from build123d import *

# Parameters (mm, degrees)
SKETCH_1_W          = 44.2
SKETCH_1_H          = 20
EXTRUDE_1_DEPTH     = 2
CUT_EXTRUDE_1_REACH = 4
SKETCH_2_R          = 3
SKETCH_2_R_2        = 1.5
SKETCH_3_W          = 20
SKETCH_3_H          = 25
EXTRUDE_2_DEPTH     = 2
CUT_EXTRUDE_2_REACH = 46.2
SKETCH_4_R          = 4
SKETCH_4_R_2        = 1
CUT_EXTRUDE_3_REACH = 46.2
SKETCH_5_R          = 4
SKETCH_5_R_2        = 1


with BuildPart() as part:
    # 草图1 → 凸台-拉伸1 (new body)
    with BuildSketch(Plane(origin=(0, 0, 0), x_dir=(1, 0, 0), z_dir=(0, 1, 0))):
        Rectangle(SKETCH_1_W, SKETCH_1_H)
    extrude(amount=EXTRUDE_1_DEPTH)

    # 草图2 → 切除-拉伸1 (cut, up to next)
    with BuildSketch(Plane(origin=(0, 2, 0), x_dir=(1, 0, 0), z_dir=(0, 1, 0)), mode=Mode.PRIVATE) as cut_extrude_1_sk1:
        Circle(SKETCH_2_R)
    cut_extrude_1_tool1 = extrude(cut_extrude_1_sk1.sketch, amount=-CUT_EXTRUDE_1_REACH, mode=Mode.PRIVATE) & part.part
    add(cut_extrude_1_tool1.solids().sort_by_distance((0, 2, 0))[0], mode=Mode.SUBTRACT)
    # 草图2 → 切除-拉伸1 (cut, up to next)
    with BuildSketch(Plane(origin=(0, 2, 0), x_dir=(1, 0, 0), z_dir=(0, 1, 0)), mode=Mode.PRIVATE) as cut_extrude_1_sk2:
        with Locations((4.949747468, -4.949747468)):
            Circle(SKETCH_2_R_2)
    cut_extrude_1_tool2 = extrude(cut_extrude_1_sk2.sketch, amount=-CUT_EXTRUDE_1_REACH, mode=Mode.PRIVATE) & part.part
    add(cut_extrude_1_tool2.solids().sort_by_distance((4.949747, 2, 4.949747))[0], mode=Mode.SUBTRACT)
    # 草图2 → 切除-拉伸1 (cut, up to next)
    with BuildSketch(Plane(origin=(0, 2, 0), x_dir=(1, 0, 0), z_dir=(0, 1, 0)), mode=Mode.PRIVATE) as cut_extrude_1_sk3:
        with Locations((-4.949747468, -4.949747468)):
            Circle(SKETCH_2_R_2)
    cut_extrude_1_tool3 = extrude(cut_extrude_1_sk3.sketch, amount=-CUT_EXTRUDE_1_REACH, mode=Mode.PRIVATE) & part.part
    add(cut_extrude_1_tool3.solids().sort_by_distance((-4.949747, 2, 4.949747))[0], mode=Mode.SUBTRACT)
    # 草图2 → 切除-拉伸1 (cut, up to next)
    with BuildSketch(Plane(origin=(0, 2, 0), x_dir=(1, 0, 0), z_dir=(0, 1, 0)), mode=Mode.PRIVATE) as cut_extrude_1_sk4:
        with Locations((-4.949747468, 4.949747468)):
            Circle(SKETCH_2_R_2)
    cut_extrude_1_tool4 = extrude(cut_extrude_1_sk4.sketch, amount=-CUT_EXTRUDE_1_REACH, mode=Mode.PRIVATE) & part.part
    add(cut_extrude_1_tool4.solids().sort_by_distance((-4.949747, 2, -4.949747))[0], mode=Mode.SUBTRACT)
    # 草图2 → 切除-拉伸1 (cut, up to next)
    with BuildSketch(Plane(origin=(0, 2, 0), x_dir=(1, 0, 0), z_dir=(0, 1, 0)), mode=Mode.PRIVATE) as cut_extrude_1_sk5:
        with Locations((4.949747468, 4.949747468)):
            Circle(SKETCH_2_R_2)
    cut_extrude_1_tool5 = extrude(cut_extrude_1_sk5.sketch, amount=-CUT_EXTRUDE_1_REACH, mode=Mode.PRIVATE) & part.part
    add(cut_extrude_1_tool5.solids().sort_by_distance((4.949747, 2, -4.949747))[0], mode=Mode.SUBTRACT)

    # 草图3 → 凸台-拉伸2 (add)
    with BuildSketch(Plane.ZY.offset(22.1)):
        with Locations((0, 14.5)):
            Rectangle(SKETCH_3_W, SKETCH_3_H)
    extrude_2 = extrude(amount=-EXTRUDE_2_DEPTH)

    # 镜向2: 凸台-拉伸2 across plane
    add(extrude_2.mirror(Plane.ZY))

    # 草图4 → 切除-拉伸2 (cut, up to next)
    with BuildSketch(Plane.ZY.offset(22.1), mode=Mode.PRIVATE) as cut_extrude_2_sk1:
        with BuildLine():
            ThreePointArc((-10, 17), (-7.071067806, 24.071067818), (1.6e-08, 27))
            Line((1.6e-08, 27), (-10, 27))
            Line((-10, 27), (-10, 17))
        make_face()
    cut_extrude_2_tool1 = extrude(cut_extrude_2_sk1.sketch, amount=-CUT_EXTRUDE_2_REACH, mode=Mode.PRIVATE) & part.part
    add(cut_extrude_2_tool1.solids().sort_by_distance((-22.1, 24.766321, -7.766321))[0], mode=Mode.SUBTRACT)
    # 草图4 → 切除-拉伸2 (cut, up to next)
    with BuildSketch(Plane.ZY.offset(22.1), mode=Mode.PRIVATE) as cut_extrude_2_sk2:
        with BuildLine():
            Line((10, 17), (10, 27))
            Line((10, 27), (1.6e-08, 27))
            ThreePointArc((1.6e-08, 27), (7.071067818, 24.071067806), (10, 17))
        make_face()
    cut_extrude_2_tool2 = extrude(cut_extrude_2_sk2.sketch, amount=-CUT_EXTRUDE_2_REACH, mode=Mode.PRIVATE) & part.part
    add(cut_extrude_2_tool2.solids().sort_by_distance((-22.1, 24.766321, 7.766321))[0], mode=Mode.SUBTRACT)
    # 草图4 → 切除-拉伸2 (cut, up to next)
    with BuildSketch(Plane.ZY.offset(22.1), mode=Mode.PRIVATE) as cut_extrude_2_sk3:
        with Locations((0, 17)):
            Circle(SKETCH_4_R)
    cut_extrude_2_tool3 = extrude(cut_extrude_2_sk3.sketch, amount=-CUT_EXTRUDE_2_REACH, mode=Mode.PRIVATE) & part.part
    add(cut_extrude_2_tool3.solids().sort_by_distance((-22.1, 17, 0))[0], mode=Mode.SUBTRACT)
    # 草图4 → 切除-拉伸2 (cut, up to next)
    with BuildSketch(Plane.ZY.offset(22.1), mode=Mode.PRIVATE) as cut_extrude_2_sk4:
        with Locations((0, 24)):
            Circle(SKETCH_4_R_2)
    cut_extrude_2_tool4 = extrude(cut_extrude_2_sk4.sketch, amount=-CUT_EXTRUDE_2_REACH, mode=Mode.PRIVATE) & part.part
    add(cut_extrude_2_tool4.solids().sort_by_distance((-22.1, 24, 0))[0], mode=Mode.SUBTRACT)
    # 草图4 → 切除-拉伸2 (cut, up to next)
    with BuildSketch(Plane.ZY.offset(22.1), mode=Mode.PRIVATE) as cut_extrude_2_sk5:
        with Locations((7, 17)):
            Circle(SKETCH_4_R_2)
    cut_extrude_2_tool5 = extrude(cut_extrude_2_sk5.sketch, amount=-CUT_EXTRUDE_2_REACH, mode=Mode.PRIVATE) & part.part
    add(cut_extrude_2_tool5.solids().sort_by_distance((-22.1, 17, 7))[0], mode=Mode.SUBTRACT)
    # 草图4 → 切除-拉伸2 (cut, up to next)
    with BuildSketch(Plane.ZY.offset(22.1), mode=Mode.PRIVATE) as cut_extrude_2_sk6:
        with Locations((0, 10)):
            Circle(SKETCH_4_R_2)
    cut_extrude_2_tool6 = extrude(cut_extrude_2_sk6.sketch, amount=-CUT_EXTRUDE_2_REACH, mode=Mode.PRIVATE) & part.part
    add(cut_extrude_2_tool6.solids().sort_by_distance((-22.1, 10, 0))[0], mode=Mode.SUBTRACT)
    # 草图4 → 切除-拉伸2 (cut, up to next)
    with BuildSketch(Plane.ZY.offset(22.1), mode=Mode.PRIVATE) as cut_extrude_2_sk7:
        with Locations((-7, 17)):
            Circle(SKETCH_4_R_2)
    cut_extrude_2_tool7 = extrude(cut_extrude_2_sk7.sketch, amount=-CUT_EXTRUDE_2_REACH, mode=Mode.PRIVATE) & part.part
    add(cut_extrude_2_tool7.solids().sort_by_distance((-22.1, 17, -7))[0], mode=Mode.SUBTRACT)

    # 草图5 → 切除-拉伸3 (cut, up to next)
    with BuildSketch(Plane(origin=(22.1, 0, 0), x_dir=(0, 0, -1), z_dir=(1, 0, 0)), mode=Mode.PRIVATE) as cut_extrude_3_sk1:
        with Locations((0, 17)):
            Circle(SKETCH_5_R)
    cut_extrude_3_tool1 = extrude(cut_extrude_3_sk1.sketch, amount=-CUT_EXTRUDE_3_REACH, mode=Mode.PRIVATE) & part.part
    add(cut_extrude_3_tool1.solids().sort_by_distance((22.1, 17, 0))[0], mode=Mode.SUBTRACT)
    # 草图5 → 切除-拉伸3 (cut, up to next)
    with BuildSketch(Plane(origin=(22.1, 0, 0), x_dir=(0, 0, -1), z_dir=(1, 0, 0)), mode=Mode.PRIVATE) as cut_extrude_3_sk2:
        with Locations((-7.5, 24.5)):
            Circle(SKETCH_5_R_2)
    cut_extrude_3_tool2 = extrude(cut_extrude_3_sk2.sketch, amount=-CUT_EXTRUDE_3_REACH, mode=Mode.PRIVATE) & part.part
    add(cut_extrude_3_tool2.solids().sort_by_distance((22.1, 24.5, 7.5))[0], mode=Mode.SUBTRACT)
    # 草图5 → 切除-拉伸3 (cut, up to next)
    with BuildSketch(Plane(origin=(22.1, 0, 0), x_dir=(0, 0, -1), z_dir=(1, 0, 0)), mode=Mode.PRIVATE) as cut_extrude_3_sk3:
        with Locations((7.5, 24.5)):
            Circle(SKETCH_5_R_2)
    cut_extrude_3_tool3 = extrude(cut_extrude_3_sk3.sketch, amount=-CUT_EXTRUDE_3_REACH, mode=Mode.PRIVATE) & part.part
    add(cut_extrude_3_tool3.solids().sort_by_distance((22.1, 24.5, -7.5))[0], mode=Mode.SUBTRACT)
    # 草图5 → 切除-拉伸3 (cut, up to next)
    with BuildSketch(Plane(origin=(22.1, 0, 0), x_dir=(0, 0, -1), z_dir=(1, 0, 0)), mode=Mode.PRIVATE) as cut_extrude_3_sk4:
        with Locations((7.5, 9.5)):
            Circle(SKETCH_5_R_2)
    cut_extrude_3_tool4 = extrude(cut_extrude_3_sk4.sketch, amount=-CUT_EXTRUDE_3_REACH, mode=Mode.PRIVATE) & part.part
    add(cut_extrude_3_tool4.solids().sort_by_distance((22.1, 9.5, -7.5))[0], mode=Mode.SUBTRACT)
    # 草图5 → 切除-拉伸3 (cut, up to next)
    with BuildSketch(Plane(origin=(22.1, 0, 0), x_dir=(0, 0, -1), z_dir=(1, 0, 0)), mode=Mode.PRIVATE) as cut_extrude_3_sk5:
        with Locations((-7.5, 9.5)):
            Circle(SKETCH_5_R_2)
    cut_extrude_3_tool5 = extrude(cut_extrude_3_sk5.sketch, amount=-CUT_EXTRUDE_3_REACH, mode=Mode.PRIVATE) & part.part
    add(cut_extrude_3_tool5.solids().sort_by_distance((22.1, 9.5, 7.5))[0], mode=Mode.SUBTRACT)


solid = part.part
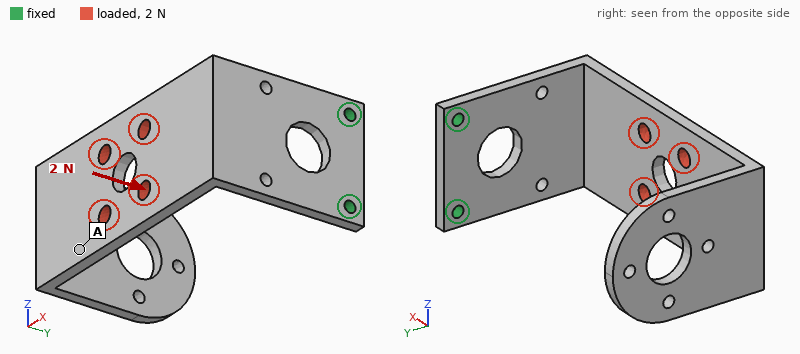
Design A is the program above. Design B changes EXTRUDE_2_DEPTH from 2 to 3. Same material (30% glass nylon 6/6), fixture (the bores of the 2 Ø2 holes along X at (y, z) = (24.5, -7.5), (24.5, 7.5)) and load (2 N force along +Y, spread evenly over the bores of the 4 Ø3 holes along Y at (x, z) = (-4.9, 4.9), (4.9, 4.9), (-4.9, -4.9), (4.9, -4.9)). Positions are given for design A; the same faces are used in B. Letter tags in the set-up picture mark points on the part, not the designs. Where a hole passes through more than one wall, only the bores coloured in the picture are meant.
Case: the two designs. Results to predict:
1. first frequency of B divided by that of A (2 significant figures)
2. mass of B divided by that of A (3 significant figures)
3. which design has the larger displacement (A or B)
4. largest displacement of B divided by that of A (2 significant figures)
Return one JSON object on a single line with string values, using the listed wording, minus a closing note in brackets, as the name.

{"first frequency of B divided by that of A": "1.2", "mass of B divided by that of A": "1.25", "which design has the larger displacement": "A", "largest displacement of B divided by that of A": "0.46"}
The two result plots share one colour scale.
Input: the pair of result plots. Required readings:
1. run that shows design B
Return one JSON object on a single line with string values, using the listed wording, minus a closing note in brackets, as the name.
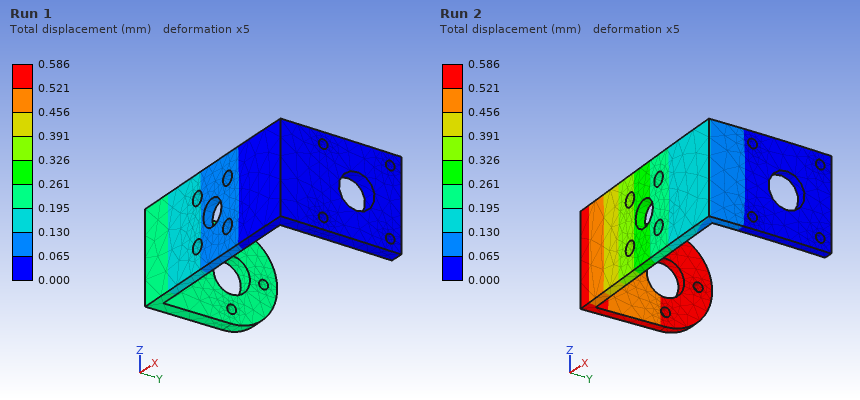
{"run that shows design B": "Run 1"}
